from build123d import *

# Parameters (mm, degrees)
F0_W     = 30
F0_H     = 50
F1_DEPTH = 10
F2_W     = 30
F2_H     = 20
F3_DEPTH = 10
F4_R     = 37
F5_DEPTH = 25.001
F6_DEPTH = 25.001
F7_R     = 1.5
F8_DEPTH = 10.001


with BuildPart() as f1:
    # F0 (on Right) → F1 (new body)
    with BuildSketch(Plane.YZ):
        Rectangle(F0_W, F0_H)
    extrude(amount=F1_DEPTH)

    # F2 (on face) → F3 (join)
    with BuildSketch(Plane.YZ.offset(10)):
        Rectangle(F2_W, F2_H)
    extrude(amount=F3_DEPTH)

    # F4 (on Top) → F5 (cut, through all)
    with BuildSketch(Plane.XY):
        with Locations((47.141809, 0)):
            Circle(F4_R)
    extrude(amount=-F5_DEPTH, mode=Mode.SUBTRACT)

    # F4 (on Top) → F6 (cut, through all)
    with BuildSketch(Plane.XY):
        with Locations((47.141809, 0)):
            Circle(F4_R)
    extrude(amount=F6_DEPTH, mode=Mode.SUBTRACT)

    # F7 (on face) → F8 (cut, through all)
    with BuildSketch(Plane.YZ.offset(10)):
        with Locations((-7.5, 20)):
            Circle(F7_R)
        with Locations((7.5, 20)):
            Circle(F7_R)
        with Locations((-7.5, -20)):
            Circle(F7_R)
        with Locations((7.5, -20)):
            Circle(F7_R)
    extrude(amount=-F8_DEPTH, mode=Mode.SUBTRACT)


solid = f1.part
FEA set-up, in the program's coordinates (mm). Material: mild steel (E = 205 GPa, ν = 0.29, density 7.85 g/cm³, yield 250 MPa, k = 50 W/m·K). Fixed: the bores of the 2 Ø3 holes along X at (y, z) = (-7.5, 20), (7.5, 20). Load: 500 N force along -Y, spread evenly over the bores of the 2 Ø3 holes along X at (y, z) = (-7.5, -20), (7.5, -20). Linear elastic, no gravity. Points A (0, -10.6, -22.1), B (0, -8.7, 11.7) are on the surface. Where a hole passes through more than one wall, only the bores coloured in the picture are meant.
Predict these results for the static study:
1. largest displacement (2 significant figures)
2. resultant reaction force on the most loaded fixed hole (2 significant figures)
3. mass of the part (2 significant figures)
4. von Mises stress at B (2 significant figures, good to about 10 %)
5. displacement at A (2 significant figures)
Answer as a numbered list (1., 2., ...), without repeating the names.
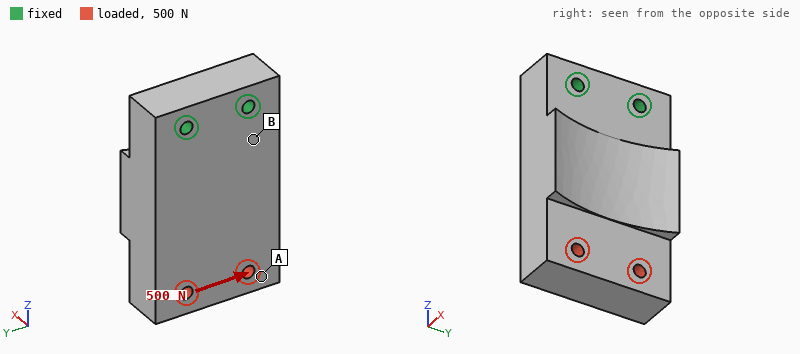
1. 5.3 µm
2. 1.2 kN
3. 120 g
4. 7.9 MPa
5. 4.8 µm
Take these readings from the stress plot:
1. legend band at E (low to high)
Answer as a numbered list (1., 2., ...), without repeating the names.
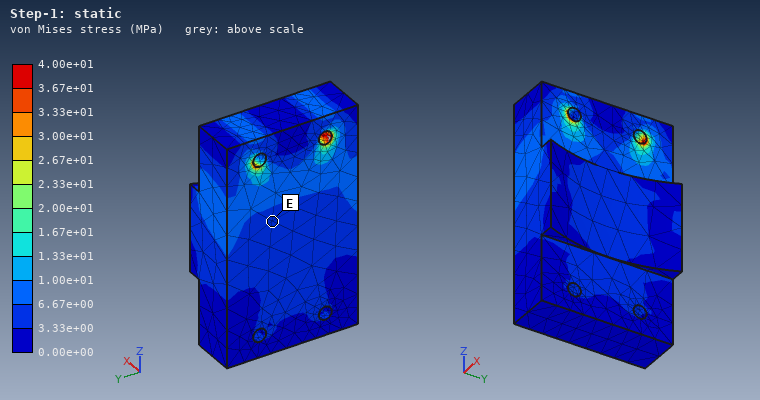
1. 3.33e+00 to 6.67e+00 MPa
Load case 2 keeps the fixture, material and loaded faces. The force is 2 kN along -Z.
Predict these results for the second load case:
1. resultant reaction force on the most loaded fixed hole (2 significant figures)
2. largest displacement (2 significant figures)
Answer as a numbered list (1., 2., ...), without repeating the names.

1. 1.0 kN
2. 1.9 µm
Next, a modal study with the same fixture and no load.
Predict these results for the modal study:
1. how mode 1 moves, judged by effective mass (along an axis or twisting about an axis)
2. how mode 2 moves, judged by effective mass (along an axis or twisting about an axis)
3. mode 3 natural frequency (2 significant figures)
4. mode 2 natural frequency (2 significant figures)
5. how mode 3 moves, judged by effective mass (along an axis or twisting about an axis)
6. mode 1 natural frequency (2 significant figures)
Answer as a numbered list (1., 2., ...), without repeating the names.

1. along X
2. along Y
3. 11 kHz
4. 8000 Hz
5. twisting about Z
6. 3800 Hz
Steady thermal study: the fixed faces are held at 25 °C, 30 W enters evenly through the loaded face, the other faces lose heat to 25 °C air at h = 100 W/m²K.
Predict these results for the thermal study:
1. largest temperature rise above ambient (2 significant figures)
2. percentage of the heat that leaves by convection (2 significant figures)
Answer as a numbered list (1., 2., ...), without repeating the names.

1. 59 K
2. 41 %
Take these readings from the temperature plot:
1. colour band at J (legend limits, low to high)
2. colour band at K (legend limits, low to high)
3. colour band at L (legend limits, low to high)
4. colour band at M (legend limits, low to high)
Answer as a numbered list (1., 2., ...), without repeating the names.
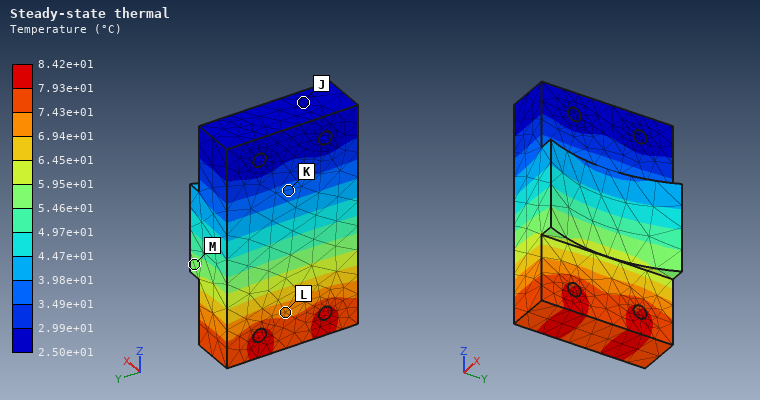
1. 2.50e+01 to 2.99e+01 °C
2. 3.49e+01 to 3.98e+01 °C
3. 6.94e+01 to 7.43e+01 °C
4. 5.46e+01 to 5.95e+01 °C
